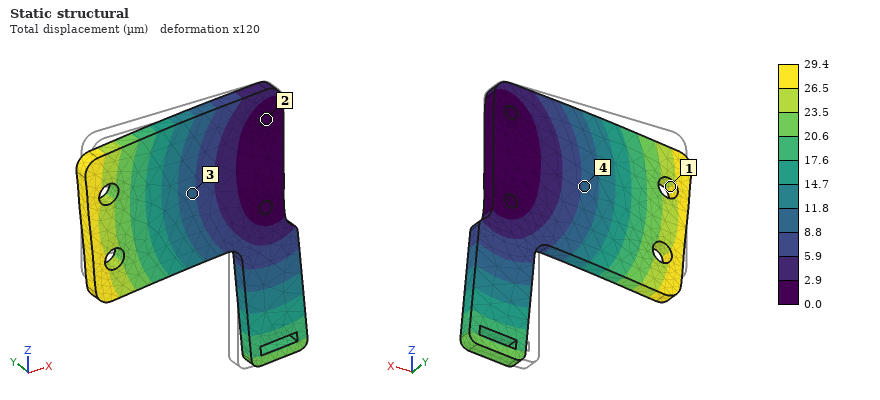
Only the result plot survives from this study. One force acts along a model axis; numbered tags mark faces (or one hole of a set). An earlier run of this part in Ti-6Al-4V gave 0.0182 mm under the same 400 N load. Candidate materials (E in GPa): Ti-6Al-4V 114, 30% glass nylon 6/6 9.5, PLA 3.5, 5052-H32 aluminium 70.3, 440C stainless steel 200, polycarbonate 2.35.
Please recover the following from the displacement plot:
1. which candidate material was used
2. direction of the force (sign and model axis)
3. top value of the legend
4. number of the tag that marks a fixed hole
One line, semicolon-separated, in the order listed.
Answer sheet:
5052-H32 aluminium; -Z; 29.4 µm; 2
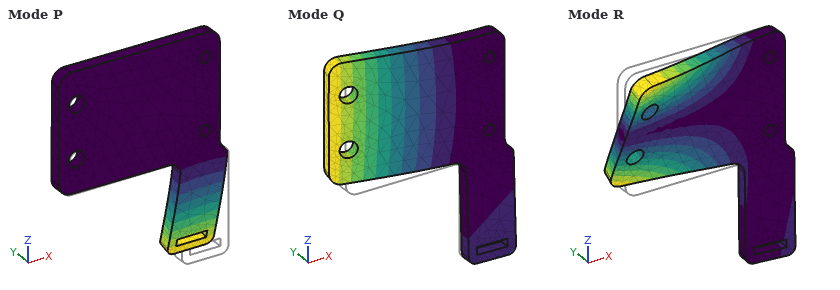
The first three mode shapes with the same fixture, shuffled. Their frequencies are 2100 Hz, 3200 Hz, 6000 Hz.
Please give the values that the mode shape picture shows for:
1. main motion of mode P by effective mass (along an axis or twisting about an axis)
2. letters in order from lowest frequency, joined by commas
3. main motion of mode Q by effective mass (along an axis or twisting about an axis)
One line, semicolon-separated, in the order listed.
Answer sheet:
along Y; Q, P, R; along Y
